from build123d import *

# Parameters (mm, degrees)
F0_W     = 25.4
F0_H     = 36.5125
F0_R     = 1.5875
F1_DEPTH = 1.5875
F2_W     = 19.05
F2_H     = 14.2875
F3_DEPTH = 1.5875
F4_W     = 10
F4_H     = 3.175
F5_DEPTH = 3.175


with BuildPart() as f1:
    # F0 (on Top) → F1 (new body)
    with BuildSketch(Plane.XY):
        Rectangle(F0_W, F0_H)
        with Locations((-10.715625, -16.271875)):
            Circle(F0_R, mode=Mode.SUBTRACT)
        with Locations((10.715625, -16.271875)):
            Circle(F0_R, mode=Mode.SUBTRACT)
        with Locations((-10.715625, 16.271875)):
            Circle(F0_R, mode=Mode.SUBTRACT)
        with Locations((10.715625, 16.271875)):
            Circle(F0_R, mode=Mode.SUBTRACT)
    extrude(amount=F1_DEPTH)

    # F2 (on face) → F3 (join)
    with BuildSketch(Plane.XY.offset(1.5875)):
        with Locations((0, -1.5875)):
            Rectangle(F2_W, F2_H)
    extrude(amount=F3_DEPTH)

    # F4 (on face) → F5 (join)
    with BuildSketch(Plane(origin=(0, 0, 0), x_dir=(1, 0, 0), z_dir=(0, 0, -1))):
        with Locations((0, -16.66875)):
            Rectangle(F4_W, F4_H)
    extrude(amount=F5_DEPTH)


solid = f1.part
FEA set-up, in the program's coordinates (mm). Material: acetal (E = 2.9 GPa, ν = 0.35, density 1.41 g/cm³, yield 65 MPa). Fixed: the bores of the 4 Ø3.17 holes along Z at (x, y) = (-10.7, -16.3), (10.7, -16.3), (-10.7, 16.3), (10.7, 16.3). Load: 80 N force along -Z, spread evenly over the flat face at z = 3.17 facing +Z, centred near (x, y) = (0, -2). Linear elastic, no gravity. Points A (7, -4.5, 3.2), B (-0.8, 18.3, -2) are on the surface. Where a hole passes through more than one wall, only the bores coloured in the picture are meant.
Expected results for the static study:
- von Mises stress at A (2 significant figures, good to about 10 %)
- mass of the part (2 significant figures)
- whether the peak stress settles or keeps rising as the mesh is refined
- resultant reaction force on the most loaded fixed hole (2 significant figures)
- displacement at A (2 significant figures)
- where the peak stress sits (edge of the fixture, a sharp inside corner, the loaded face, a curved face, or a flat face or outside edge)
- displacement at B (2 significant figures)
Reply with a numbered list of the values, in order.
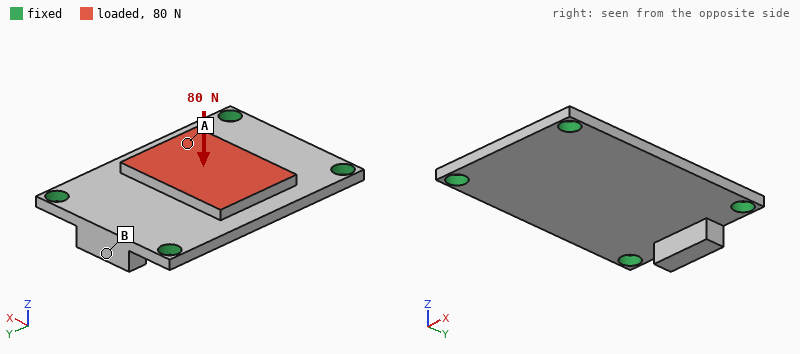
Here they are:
1. 7.4 MPa
2. 2.8 g
3. keeps rising
4. 29 N
5. 0.21 mm
6. edge of the fixture
7. 0.063 mm
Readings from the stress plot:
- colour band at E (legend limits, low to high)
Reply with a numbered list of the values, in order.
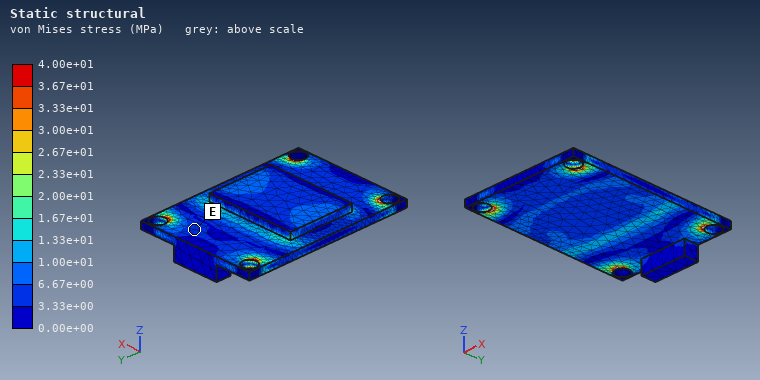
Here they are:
1. 3.33e+00 to 6.67e+00 MPa
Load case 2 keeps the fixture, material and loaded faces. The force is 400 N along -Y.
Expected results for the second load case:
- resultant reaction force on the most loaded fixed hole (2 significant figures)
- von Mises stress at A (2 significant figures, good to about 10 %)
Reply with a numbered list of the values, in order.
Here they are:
1. 110 N
2. 4.3 MPa
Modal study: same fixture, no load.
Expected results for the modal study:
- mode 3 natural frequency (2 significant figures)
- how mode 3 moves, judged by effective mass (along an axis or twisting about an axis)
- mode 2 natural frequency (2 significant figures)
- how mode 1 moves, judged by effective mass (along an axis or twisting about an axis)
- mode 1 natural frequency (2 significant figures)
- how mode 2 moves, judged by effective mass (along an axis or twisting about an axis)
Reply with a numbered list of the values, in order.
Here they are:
1. 5400 Hz
2. twisting about X
3. 3400 Hz
4. along Z
5. 2300 Hz
6. twisting about Y
